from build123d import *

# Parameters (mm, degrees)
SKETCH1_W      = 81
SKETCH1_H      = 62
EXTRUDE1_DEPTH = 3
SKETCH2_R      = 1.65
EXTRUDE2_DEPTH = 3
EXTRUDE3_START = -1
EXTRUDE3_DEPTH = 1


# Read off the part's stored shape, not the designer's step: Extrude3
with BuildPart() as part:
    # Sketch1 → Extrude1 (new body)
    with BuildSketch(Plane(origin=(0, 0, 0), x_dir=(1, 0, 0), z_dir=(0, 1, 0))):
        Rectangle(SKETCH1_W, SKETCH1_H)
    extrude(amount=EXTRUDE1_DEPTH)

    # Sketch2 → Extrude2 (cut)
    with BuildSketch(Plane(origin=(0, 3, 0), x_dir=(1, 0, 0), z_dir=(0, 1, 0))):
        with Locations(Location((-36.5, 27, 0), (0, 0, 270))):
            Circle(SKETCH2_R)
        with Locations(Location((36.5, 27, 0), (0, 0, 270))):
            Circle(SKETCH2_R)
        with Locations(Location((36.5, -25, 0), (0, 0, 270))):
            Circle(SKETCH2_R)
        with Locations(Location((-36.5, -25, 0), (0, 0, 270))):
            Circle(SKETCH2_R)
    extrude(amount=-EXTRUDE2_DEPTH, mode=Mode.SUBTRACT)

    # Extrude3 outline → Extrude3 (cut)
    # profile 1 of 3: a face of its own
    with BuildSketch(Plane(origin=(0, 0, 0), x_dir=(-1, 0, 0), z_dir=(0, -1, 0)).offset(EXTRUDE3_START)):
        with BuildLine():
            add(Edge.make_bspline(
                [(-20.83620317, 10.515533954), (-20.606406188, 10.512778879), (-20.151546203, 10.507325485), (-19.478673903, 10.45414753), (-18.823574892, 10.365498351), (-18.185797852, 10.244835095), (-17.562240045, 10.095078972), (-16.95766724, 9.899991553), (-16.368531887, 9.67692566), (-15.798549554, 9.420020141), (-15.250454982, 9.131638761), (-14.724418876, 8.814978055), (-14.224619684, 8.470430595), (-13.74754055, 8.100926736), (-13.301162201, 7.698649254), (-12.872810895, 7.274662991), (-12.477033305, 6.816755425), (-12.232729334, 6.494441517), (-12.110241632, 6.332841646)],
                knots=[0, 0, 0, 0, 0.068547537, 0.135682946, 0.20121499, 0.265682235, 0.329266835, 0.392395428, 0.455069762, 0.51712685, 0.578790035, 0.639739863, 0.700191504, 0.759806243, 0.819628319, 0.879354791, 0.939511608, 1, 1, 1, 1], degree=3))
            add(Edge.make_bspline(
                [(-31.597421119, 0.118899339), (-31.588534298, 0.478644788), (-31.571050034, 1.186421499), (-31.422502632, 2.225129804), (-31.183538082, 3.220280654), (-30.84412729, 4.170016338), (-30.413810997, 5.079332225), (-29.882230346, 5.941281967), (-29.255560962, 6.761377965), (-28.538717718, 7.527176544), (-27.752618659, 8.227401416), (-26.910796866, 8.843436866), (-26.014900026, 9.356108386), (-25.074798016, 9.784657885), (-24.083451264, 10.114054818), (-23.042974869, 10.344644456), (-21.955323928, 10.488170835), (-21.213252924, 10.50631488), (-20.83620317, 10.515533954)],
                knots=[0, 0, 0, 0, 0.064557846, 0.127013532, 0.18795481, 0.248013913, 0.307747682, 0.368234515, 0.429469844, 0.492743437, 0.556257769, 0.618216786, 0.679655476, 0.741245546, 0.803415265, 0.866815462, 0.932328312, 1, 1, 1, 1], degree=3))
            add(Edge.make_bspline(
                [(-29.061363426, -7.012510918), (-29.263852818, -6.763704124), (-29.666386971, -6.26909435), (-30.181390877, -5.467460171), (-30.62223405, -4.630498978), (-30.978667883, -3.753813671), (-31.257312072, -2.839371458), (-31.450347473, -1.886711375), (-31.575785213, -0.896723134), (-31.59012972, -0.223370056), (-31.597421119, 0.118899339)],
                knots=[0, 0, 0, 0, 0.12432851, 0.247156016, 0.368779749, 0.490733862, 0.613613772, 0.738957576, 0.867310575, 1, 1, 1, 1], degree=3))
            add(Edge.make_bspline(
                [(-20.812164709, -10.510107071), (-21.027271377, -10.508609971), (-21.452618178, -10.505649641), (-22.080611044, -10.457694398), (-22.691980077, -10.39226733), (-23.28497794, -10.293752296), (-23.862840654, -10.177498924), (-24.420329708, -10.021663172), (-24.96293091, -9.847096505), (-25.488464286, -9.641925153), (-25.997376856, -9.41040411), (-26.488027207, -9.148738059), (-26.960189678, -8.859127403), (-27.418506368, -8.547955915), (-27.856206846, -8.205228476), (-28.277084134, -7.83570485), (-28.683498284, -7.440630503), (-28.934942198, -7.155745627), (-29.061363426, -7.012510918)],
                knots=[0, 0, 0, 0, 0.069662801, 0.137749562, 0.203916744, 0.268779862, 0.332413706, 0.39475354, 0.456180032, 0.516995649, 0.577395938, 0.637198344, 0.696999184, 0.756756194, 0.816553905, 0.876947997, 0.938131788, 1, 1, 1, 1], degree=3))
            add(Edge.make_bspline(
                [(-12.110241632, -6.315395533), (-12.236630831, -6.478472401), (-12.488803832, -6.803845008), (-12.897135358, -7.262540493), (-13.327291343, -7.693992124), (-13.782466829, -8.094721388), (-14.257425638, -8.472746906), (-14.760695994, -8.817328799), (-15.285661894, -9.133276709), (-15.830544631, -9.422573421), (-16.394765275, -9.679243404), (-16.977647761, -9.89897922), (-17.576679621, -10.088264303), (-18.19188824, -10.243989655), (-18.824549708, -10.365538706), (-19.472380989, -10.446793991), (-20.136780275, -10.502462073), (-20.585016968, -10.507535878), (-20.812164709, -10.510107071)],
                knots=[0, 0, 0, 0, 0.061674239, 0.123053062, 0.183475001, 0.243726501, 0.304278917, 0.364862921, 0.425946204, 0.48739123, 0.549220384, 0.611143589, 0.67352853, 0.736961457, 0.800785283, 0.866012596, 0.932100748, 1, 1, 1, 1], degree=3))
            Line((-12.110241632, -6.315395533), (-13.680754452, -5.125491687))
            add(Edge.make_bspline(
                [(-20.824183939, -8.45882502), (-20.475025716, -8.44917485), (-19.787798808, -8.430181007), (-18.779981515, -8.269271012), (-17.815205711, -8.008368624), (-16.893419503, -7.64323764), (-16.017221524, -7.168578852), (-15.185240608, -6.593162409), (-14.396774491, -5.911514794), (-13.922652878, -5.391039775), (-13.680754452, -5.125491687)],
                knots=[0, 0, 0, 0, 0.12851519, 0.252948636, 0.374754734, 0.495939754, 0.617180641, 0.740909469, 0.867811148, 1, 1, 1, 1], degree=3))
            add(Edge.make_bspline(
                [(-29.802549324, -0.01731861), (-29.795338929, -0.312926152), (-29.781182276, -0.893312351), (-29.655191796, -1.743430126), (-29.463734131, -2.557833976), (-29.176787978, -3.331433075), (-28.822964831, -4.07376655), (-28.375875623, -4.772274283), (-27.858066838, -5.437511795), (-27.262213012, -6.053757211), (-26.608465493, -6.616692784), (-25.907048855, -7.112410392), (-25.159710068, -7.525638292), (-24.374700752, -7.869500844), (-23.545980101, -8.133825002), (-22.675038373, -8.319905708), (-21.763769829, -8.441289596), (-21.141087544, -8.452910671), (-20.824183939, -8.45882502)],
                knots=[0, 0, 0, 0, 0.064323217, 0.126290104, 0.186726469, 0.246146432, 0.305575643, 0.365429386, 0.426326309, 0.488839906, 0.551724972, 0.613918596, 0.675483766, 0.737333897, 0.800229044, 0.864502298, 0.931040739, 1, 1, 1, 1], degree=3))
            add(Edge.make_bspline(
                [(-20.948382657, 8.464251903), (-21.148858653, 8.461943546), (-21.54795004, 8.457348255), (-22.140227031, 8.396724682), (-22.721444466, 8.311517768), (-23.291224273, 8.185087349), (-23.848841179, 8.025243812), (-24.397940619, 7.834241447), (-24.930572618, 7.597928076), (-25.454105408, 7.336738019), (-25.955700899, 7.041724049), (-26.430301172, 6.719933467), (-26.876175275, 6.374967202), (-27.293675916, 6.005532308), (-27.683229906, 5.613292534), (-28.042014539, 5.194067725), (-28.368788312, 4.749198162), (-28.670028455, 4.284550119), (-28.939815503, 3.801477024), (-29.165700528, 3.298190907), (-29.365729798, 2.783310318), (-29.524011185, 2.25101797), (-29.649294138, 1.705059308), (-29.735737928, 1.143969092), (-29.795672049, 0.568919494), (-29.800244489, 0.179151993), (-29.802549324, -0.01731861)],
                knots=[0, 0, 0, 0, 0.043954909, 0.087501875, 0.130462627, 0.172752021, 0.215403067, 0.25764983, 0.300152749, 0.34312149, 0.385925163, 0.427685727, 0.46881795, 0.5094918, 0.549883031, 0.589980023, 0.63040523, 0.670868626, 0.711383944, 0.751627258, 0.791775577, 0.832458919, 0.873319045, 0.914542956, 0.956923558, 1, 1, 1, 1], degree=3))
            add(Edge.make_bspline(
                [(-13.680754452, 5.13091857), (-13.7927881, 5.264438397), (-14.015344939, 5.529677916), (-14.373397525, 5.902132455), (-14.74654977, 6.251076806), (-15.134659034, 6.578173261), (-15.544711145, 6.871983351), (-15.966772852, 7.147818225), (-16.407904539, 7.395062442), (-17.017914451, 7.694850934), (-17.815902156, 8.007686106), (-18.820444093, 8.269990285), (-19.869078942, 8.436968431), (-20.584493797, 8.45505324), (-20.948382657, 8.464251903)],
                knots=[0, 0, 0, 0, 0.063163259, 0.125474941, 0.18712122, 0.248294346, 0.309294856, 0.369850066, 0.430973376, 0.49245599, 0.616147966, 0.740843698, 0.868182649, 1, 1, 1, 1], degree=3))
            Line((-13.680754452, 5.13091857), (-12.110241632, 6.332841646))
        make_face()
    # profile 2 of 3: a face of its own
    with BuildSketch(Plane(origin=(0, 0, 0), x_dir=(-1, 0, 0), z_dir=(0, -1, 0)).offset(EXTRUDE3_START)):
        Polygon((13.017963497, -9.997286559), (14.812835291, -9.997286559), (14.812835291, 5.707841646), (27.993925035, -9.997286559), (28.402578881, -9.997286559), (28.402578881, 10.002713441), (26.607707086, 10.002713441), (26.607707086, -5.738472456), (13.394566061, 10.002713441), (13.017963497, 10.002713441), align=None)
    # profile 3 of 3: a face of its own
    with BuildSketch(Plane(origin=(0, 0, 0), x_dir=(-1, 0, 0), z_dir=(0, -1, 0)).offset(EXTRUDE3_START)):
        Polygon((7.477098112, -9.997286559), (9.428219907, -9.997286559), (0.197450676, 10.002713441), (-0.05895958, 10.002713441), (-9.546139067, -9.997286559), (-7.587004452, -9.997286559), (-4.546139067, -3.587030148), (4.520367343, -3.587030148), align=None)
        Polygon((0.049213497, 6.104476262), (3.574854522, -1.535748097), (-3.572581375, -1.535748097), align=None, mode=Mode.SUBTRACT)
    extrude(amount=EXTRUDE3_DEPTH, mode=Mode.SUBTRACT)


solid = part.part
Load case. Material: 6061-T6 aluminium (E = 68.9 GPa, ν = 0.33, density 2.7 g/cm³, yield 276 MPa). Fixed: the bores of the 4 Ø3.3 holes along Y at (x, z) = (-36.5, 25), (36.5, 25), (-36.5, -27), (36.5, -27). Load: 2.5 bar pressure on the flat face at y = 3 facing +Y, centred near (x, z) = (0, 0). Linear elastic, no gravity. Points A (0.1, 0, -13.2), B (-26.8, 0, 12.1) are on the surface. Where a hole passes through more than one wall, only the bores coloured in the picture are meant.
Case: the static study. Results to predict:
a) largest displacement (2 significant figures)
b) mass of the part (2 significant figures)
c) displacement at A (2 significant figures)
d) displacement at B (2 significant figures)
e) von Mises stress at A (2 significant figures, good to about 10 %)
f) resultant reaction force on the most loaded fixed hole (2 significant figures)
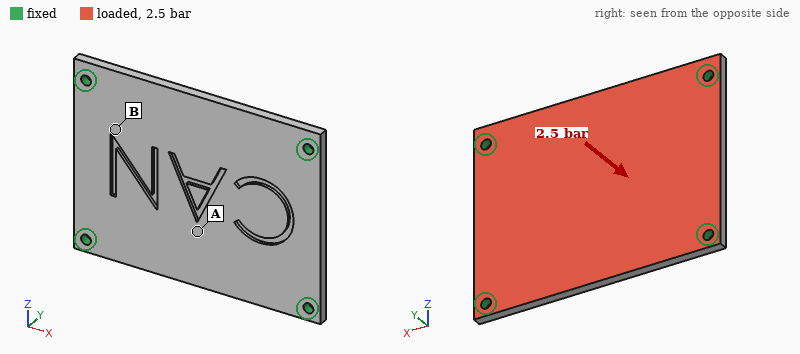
0.22 mm
40 g
0.21 mm
0.085 mm
51 MPa
330 N
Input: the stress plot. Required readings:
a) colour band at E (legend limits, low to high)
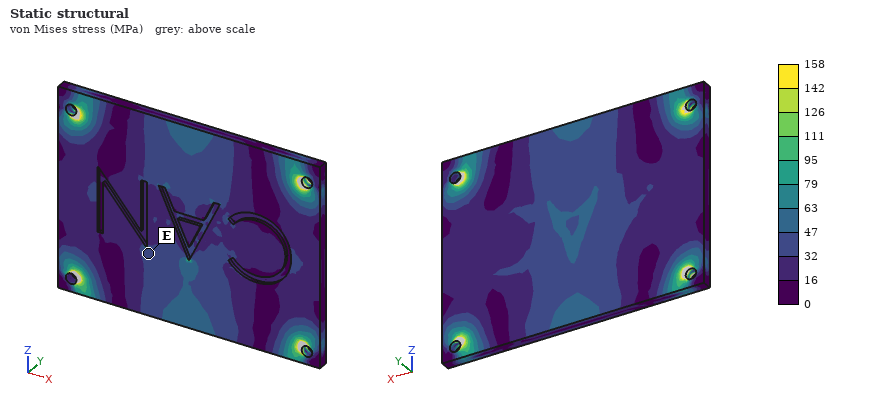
32 to 47 MPa
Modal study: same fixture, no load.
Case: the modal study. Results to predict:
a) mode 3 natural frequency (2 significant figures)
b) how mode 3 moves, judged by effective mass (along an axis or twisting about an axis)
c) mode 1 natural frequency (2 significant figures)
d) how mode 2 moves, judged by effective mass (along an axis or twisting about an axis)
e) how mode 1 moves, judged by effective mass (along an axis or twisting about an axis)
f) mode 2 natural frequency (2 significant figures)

5200 Hz
twisting about Z
2300 Hz
twisting about X
along Y
3600 Hz
